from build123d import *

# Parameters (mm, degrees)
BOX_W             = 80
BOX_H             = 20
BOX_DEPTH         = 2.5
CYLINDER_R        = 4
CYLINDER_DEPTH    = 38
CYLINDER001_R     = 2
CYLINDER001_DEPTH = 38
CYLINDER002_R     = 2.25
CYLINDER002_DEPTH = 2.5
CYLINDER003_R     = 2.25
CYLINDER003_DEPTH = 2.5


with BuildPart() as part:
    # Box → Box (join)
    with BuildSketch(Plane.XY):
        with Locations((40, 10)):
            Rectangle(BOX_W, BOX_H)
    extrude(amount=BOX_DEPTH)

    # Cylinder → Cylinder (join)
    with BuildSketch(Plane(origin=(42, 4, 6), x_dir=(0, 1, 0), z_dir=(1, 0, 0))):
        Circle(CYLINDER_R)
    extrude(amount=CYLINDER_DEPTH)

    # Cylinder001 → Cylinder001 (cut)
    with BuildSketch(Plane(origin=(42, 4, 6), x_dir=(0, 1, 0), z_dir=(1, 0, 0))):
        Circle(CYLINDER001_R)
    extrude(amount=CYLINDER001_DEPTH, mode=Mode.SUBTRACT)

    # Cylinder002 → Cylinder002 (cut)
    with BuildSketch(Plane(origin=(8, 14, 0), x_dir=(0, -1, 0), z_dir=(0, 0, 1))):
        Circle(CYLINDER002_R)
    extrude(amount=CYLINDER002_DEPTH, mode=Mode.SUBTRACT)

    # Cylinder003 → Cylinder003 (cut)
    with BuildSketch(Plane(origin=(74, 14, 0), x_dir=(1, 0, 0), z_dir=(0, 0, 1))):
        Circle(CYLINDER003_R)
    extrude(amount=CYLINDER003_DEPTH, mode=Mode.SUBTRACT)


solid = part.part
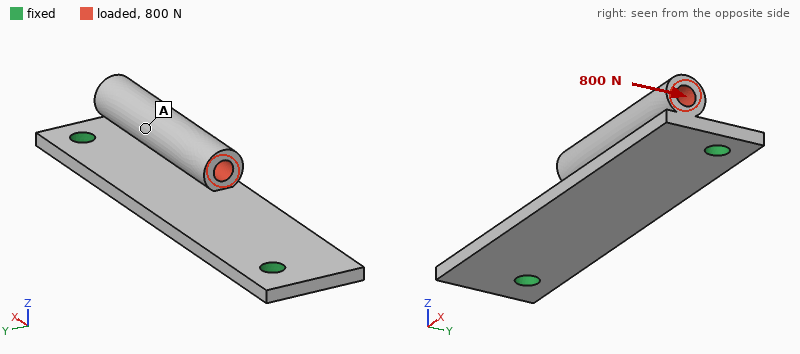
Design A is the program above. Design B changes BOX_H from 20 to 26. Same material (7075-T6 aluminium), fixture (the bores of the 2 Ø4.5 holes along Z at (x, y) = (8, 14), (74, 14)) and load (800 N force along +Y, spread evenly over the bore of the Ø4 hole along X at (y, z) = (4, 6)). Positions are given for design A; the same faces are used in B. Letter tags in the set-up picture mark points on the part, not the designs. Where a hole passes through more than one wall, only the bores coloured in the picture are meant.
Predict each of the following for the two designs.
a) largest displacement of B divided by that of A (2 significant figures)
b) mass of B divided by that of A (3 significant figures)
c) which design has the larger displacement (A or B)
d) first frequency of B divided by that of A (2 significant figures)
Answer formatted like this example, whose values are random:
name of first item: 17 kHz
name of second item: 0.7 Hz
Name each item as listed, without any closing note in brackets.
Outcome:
largest displacement of B divided by that of A: 0.92
mass of B divided by that of A: 1.23
which design has the larger displacement: A
first frequency of B divided by that of A: 0.96
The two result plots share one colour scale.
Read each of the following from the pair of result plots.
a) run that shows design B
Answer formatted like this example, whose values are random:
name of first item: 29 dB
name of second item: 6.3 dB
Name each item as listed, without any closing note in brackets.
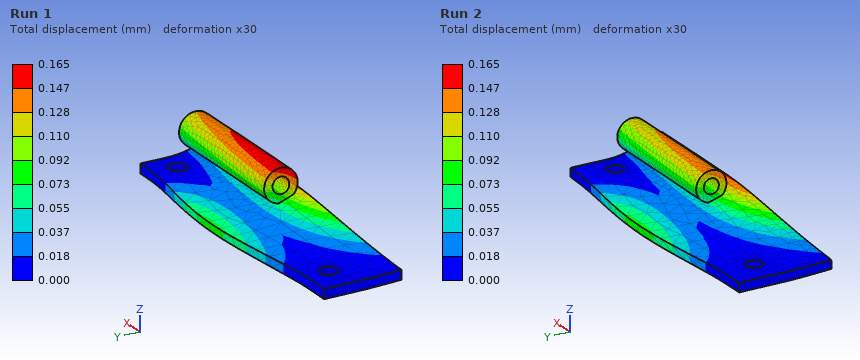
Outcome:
run that shows design B: Run 2
